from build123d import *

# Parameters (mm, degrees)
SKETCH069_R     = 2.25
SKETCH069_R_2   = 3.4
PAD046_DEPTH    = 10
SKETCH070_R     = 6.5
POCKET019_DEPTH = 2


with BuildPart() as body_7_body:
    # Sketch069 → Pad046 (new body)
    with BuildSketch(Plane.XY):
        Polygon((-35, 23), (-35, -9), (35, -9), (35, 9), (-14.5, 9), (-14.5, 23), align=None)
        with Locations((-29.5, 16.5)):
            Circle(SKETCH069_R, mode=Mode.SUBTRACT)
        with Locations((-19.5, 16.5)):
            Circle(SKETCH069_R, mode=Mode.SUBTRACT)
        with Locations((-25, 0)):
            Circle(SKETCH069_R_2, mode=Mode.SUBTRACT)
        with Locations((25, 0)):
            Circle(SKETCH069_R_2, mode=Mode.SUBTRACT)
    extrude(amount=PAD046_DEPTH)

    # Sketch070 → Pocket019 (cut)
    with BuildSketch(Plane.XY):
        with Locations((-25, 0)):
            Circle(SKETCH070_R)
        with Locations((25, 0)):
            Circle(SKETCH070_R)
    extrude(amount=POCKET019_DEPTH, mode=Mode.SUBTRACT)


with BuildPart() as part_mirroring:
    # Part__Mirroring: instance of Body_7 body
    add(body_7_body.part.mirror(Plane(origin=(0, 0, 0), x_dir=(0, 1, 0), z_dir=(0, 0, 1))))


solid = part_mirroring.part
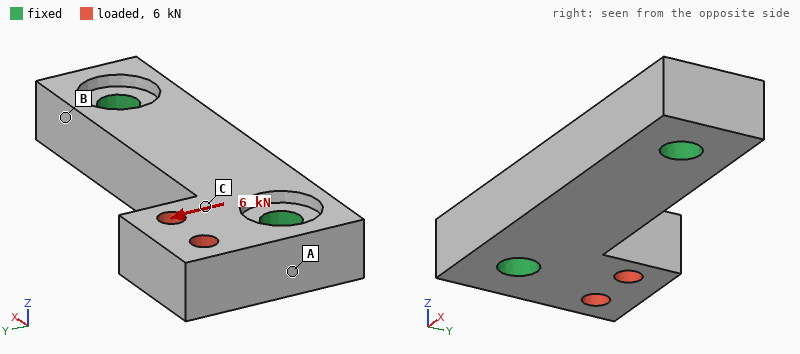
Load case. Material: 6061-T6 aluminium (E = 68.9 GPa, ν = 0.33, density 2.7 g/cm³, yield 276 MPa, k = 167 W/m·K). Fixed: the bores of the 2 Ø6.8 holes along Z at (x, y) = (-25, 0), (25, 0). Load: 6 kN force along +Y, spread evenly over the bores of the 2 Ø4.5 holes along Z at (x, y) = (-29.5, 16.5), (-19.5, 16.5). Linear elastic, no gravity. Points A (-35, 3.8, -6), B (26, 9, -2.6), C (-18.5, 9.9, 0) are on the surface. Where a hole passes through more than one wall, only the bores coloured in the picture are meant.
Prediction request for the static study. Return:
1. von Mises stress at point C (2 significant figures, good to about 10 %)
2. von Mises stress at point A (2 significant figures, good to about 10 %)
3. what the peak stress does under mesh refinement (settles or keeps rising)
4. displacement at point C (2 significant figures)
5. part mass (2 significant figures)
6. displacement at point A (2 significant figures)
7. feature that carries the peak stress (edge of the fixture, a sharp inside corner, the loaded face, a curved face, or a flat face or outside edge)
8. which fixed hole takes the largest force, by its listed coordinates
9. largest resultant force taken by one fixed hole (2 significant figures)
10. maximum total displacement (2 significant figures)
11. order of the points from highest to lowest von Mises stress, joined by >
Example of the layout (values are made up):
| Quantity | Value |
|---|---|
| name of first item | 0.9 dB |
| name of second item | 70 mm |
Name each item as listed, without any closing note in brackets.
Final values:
| Quantity | Value |
|---|---|
| von Mises stress at point C | 26 MPa |
| von Mises stress at point A | 14 MPa |
| what the peak stress does under mesh refinement | keeps rising |
| displacement at point C | 7.8 µm |
| part mass | 38 g |
| displacement at point A | 4.9 µm |
| feature that carries the peak stress | edge of the fixture |
| which fixed hole takes the largest force, by its listed coordinates | (-25, 0) |
| largest resultant force taken by one fixed hole | 5.9 kN |
| maximum total displacement | 15 µm |
| order of the points from highest to lowest von Mises stress, joined by > | C > A > B |
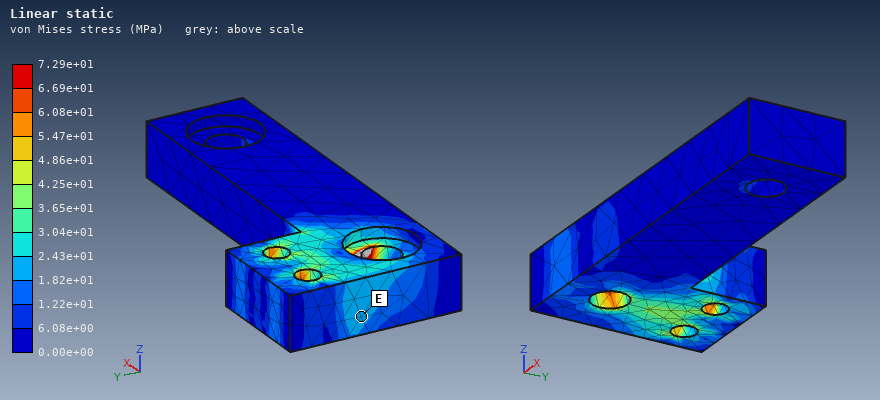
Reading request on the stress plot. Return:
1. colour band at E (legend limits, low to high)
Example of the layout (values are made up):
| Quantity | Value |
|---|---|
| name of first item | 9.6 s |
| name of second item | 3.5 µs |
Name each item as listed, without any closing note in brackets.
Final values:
| Quantity | Value |
|---|---|
| colour band at E | 1.82e+01 to 2.43e+01 MPa |
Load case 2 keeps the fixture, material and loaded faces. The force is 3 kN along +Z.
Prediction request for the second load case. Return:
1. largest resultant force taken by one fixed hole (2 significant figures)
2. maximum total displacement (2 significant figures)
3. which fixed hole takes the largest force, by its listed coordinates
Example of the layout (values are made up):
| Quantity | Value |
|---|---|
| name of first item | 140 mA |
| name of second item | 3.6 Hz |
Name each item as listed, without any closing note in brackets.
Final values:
| Quantity | Value |
|---|---|
| largest resultant force taken by one fixed hole | 3.0 kN |
| maximum total displacement | 86 µm |
| which fixed hole takes the largest force, by its listed coordinates | (-25, 0) |
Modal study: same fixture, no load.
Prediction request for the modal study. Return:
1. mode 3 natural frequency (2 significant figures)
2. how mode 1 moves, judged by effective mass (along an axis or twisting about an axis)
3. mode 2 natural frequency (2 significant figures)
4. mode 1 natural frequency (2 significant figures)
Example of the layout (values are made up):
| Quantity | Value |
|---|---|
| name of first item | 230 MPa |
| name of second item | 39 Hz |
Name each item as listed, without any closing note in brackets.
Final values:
| Quantity | Value |
|---|---|
| mode 3 natural frequency | 17 kHz |
| how mode 1 moves, judged by effective mass | along Z |
| mode 2 natural frequency | 16 kHz |
| mode 1 natural frequency | 13 kHz |
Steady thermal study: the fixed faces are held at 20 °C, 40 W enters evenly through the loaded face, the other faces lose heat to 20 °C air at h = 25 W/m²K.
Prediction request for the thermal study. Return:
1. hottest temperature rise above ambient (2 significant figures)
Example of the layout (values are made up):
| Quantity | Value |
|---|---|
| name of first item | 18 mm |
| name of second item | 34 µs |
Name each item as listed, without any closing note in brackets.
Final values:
| Quantity | Value |
|---|---|
| hottest temperature rise above ambient | 22 K |
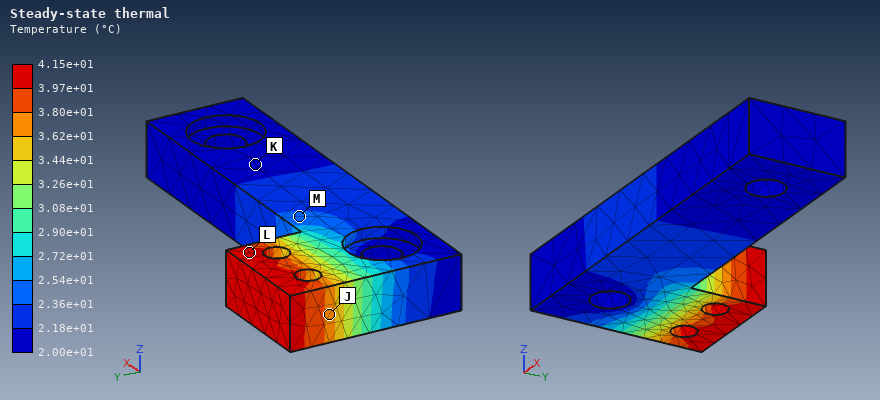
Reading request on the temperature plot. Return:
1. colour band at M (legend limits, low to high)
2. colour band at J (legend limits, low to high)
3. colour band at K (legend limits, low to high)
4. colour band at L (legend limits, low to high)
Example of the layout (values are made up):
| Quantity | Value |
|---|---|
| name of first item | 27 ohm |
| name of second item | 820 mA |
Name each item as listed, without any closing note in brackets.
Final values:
| Quantity | Value |
|---|---|
| colour band at M | 2.36e+01 to 2.54e+01 °C |
| colour band at J | 3.62e+01 to 3.80e+01 °C |
| colour band at K | 2.00e+01 to 2.18e+01 °C |
| colour band at L | 3.97e+01 to 4.15e+01 °C |
